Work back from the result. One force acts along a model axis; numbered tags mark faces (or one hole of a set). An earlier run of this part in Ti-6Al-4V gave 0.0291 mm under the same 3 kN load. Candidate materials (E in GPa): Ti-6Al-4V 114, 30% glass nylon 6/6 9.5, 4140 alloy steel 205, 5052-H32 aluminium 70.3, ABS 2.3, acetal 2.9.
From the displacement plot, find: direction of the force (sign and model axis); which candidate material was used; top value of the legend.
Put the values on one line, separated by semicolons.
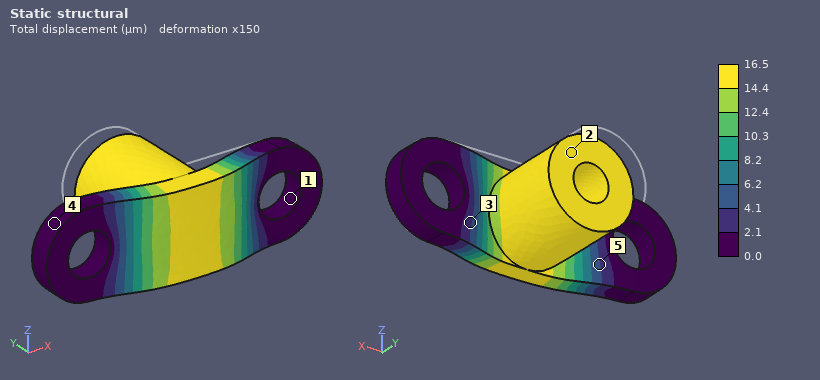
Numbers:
-Y; 4140 alloy steel; 16.5 µm
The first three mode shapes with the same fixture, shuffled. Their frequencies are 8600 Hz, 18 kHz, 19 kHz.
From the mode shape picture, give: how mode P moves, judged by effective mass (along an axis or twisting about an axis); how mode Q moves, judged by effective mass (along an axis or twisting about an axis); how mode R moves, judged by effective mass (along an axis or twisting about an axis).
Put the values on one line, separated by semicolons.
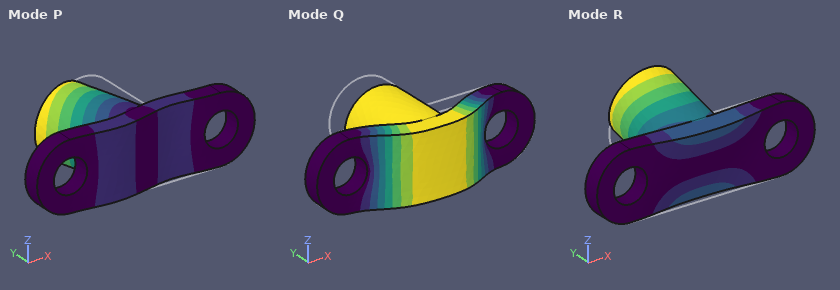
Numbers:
along X; along Y; along Z
